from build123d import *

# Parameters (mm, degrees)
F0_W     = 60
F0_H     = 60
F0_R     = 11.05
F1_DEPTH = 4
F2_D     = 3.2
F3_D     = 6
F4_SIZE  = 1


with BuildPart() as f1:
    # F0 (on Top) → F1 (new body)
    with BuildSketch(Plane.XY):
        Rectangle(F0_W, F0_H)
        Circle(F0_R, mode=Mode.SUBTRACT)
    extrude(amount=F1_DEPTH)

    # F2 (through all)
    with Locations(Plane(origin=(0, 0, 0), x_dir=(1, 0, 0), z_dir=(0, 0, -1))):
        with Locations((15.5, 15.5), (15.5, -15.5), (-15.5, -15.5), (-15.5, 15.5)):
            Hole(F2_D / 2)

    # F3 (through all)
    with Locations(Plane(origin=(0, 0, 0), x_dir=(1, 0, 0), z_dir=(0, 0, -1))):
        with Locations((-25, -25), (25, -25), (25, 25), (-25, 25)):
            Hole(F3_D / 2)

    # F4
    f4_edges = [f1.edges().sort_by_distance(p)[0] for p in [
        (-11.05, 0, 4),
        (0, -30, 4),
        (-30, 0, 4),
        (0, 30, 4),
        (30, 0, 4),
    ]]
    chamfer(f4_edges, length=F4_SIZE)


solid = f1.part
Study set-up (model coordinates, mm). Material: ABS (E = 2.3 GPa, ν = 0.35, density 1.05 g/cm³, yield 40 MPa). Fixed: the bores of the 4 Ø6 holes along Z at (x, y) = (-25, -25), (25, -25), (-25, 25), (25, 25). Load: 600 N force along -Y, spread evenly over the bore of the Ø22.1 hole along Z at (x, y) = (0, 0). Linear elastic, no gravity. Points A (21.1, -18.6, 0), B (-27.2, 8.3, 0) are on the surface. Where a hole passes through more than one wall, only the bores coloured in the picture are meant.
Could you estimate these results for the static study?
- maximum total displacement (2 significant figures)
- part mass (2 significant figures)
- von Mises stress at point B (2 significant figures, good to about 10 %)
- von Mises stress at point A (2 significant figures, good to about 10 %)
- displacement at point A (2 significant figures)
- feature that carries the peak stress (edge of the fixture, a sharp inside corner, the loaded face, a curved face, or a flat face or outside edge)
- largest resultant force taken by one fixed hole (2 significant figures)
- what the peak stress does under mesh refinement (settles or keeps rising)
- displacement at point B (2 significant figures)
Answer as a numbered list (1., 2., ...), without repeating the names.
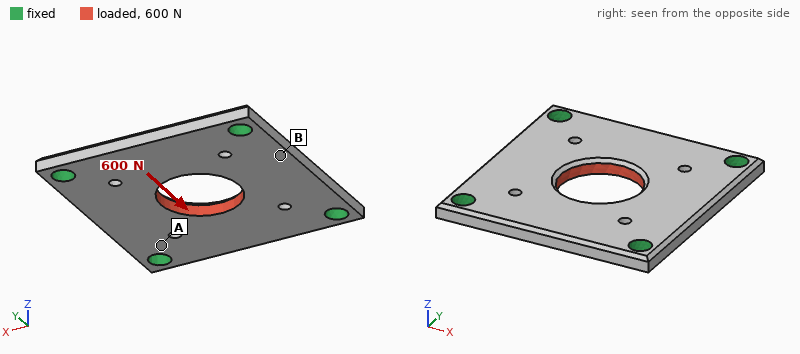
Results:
1. 49 µm
2. 13 g
3. 1.1 MPa
4. 3.4 MPa
5. 8.6 µm
6. edge of the fixture
7. 170 N
8. keeps rising
9. 11 µm
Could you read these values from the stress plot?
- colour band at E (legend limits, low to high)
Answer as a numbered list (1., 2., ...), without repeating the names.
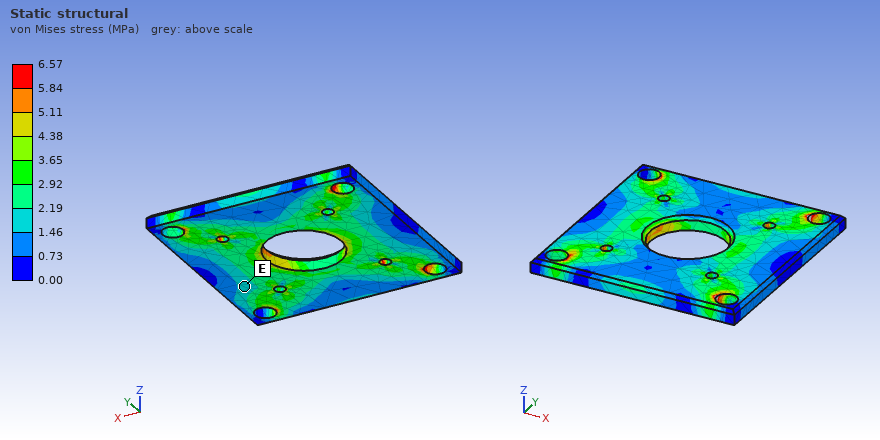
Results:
1. 1.46 to 2.19 MPa
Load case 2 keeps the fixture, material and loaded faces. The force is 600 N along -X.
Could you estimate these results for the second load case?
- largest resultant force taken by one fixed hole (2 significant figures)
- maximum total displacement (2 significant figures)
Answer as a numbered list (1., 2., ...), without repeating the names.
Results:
1. 170 N
2. 49 µm
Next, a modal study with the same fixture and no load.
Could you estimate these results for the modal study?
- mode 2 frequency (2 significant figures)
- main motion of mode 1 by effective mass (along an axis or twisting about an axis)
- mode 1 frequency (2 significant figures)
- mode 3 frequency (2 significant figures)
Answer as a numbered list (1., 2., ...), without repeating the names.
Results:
1. 2800 Hz
2. along Z
3. 1900 Hz
4. 2800 Hz
